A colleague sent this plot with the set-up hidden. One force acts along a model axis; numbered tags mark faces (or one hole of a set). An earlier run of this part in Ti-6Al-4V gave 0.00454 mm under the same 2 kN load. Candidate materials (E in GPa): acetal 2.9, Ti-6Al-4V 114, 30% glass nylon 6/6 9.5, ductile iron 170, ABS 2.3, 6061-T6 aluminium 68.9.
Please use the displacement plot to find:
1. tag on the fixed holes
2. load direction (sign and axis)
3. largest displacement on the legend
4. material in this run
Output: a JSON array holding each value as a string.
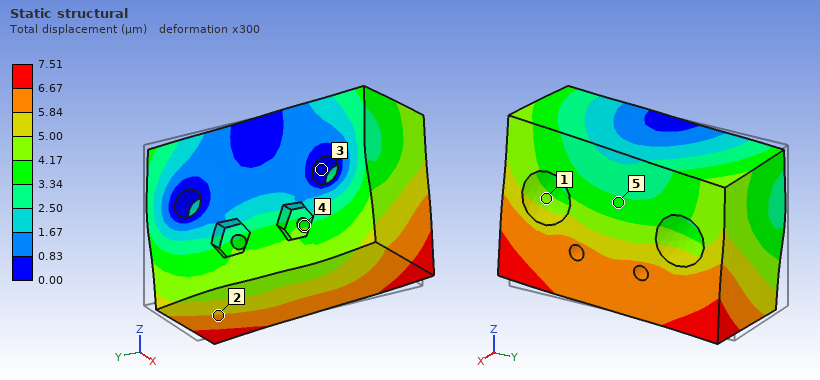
["3", "-Y", "7.51 µm", "6061-T6 aluminium"]
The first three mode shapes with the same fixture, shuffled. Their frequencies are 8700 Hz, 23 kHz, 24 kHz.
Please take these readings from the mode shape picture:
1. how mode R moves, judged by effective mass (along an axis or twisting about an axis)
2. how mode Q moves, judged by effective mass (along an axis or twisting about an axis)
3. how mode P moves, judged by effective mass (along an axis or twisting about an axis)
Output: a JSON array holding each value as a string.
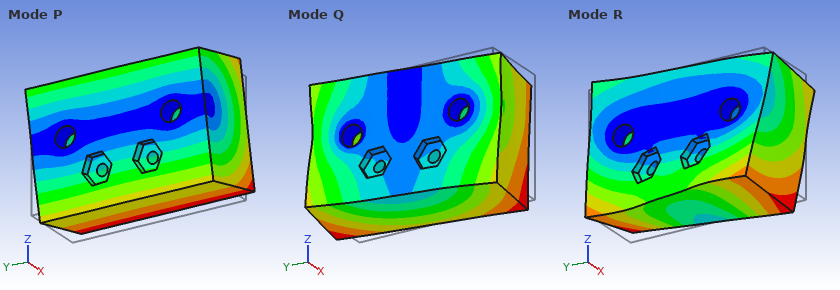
["twisting about X", "along Y", "along Z"]
